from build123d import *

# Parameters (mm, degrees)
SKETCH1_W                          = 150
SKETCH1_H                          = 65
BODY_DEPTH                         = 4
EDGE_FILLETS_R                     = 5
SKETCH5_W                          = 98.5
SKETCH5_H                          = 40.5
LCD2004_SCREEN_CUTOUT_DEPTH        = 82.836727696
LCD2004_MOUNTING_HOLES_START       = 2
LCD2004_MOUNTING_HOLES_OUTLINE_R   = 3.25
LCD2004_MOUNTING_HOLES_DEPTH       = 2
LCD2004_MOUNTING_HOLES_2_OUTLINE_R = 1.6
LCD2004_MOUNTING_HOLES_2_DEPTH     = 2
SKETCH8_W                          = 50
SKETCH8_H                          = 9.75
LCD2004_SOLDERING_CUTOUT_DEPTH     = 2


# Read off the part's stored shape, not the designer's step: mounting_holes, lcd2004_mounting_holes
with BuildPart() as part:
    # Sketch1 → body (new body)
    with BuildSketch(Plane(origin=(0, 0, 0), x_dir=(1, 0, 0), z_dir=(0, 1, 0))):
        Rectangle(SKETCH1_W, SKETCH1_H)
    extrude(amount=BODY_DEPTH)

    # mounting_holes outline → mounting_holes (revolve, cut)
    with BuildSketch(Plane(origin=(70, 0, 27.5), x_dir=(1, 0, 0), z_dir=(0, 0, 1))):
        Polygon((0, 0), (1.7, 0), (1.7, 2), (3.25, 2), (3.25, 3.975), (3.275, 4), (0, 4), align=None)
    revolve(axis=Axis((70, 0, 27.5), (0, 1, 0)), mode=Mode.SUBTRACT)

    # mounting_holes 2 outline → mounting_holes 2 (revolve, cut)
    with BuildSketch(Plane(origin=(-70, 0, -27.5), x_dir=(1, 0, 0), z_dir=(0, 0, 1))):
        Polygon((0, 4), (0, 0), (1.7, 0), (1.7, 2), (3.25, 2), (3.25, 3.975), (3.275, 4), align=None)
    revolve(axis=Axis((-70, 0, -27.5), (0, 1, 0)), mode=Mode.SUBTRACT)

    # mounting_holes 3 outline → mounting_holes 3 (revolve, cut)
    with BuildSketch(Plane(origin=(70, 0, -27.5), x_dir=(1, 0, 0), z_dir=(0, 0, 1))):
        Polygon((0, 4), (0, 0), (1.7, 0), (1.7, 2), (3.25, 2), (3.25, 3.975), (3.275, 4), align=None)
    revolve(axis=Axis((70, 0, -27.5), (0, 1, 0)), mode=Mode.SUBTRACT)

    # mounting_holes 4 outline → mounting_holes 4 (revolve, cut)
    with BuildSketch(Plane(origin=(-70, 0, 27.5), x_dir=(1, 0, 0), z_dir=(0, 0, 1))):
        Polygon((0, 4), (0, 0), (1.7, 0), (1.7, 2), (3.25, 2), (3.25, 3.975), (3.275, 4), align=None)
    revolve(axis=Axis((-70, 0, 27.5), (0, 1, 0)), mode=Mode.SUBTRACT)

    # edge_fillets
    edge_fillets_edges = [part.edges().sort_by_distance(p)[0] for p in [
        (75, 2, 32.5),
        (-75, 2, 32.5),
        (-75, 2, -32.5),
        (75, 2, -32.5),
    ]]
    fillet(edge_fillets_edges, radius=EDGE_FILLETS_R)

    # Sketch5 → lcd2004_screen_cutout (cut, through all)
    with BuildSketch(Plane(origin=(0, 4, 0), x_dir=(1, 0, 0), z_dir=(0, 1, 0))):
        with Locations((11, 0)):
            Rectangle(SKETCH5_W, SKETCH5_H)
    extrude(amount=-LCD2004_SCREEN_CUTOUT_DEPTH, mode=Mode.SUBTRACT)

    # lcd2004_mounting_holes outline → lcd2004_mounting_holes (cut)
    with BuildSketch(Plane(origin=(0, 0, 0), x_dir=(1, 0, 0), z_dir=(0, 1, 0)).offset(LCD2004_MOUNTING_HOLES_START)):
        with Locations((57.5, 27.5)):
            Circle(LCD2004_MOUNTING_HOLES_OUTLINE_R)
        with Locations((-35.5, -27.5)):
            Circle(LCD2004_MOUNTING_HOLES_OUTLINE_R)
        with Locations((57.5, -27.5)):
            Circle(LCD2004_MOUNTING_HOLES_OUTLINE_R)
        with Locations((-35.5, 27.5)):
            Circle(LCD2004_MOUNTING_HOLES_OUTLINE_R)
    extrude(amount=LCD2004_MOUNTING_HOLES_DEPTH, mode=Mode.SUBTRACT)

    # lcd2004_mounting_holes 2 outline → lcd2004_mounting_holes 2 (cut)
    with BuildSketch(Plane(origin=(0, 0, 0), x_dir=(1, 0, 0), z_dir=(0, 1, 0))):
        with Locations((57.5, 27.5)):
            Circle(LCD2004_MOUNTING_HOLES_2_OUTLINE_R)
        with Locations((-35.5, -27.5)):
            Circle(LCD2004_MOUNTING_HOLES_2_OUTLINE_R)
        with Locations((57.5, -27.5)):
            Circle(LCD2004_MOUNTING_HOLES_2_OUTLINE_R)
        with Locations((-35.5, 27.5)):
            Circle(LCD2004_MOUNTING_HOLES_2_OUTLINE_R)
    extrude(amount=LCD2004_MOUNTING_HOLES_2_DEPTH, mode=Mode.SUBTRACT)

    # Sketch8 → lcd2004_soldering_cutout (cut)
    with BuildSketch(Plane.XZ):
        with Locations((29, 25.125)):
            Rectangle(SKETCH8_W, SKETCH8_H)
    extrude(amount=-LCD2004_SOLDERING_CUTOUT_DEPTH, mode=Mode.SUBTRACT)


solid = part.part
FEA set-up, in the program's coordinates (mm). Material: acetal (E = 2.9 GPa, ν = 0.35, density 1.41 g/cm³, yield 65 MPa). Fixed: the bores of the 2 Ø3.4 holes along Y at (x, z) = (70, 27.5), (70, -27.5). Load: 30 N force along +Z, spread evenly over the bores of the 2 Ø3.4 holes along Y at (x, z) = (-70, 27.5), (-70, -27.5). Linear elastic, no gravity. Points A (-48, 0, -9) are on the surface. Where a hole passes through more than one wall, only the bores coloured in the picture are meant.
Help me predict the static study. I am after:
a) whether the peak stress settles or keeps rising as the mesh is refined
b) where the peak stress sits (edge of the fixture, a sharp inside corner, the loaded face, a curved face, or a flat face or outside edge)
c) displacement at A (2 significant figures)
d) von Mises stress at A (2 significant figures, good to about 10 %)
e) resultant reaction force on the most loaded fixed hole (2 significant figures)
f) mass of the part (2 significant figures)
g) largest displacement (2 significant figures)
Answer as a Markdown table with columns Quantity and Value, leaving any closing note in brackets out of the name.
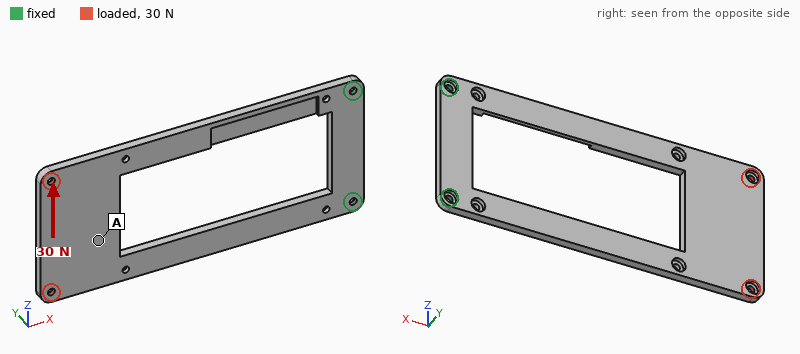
| Quantity | Value |
|---|---|
| whether the peak stress settles or keeps rising as the mesh is refined | keeps rising |
| where the peak stress sits | edge of the fixture |
| displacement at A | 1.4 mm |
| von Mises stress at A | 1.2 MPa |
| resultant reaction force on the most loaded fixed hole | 73 N |
| mass of the part | 30 g |
| largest displacement | 1.6 mm |
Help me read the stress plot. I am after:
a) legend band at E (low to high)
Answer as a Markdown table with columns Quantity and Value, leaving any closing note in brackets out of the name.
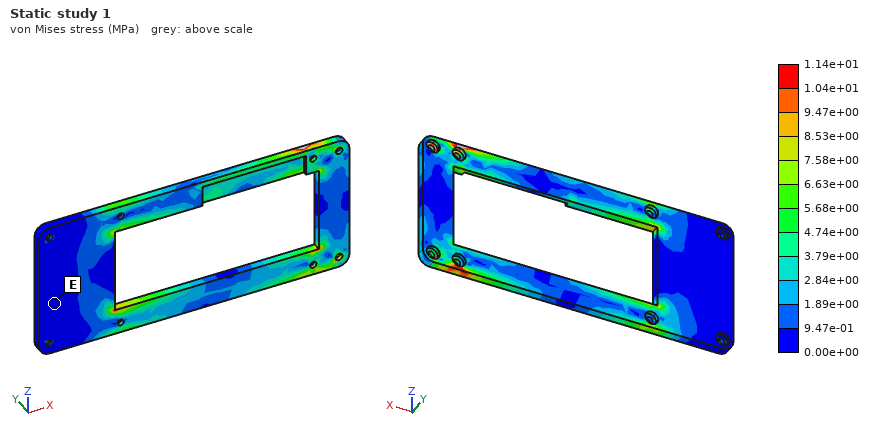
| Quantity | Value |
|---|---|
| legend band at E | 0.00e+00 to 9.47e-01 MPa |
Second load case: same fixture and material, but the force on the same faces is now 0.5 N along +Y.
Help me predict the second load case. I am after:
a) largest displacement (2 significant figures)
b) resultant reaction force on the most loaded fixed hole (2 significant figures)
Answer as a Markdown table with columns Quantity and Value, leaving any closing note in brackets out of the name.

| Quantity | Value |
|---|---|
| largest displacement | 1.9 mm |
| resultant reaction force on the most loaded fixed hole | 0.75 N |
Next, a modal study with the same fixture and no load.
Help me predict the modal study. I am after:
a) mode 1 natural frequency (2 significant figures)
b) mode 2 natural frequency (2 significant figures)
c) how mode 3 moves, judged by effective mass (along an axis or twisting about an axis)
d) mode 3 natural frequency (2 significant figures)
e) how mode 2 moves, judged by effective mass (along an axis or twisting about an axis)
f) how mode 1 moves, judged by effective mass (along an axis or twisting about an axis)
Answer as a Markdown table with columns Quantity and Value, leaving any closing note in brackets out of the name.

| Quantity | Value |
|---|---|
| mode 1 natural frequency | 25 Hz |
| mode 2 natural frequency | 110 Hz |
| how mode 3 moves, judged by effective mass | along Z |
| mode 3 natural frequency | 180 Hz |
| how mode 2 moves, judged by effective mass | twisting about X |
| how mode 1 moves, judged by effective mass | along Y |
